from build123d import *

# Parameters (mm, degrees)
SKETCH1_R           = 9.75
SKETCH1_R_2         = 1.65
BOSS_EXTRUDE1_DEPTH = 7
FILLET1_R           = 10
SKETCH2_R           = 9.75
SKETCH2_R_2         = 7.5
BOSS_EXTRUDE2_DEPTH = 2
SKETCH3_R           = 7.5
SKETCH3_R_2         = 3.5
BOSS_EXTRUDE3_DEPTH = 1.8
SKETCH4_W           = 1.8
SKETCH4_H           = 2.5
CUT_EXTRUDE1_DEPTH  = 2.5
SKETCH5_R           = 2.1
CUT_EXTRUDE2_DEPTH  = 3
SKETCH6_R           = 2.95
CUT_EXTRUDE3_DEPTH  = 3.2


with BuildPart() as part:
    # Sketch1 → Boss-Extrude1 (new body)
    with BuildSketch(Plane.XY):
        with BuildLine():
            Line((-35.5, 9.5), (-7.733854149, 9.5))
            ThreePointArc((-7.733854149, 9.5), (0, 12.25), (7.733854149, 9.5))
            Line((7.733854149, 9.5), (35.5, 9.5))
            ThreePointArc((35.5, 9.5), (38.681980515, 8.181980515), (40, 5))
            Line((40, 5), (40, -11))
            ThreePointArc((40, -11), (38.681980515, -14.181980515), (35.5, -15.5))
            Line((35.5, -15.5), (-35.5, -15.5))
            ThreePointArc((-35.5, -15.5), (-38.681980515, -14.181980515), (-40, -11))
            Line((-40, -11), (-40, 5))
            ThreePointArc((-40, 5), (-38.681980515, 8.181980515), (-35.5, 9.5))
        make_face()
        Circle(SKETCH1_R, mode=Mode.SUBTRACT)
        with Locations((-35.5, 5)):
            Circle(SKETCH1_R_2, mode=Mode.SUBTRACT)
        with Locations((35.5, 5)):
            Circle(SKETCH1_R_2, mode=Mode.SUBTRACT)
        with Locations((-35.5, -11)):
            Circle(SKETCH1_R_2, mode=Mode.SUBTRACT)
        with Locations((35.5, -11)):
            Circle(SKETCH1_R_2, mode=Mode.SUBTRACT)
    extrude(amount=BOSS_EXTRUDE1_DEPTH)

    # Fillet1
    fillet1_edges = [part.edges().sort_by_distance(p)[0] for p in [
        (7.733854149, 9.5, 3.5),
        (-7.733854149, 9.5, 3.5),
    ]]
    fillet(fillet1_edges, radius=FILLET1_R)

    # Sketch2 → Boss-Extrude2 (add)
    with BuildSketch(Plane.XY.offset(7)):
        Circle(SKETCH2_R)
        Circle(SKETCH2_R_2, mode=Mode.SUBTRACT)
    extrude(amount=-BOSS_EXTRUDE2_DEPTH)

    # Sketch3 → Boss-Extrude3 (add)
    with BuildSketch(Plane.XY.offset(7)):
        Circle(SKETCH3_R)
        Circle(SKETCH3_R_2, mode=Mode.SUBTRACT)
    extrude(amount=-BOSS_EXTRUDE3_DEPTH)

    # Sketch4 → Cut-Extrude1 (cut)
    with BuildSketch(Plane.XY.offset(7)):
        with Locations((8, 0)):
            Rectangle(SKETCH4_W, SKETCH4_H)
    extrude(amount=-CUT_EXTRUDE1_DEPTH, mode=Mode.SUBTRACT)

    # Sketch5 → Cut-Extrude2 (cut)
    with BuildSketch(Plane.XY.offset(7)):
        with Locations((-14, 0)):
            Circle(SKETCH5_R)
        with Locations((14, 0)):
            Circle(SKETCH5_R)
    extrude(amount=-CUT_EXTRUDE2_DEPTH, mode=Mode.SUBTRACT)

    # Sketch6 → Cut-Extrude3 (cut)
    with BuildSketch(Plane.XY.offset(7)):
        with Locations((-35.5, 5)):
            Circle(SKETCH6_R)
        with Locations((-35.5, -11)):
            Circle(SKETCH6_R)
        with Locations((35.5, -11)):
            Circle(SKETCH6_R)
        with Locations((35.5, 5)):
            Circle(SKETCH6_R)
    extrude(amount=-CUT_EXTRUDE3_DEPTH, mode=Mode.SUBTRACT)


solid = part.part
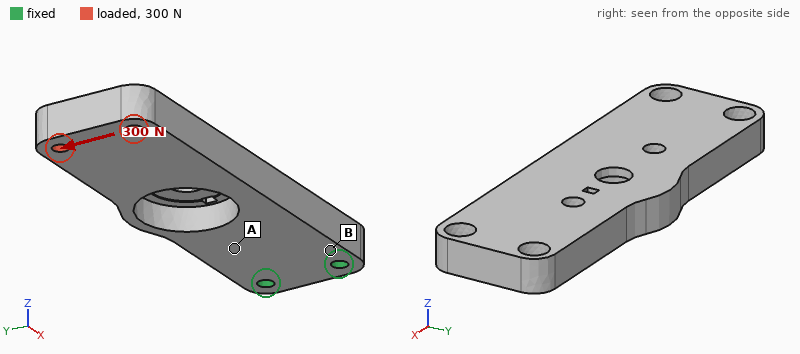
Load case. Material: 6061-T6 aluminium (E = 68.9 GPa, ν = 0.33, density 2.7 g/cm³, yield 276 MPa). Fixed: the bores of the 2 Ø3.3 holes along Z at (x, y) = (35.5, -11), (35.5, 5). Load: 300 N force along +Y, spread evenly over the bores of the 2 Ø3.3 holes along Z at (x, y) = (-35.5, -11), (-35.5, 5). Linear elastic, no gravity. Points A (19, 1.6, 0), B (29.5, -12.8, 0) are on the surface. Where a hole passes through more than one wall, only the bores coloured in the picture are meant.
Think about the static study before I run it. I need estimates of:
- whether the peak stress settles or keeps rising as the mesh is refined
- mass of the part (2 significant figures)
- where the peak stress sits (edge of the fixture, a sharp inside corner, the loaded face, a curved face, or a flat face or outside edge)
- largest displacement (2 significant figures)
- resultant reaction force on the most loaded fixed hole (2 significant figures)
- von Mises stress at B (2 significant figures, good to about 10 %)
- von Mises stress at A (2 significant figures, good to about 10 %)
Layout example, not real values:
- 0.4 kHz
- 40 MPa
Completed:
- keeps rising
- 32 g
- edge of the fixture
- 0.11 mm
- 1.2 kN
- 29 MPa
- 14 MPa
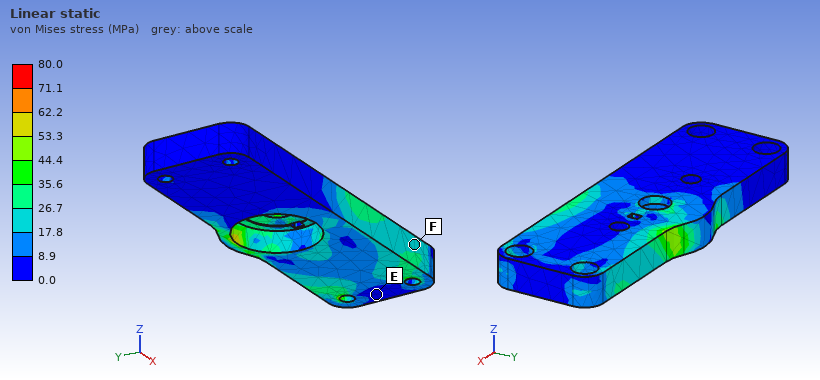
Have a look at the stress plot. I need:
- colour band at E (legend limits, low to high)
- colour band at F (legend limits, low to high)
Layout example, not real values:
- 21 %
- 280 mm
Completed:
- 0.0 to 8.9 MPa
- 17.8 to 26.7 MPa
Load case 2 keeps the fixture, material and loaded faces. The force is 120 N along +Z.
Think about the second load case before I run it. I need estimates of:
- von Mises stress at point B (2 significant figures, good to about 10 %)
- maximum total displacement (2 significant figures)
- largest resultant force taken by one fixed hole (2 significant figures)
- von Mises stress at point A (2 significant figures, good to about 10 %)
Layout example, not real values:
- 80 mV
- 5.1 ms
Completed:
- 44 MPa
- 0.54 mm
- 82 N
- 27 MPa
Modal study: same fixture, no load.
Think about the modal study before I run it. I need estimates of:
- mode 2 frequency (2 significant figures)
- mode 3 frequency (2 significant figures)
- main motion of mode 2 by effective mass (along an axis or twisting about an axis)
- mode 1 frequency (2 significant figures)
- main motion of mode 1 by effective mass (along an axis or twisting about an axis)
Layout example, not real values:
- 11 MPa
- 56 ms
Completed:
- 2900 Hz
- 4700 Hz
- along Y
- 810 Hz
- along Z
